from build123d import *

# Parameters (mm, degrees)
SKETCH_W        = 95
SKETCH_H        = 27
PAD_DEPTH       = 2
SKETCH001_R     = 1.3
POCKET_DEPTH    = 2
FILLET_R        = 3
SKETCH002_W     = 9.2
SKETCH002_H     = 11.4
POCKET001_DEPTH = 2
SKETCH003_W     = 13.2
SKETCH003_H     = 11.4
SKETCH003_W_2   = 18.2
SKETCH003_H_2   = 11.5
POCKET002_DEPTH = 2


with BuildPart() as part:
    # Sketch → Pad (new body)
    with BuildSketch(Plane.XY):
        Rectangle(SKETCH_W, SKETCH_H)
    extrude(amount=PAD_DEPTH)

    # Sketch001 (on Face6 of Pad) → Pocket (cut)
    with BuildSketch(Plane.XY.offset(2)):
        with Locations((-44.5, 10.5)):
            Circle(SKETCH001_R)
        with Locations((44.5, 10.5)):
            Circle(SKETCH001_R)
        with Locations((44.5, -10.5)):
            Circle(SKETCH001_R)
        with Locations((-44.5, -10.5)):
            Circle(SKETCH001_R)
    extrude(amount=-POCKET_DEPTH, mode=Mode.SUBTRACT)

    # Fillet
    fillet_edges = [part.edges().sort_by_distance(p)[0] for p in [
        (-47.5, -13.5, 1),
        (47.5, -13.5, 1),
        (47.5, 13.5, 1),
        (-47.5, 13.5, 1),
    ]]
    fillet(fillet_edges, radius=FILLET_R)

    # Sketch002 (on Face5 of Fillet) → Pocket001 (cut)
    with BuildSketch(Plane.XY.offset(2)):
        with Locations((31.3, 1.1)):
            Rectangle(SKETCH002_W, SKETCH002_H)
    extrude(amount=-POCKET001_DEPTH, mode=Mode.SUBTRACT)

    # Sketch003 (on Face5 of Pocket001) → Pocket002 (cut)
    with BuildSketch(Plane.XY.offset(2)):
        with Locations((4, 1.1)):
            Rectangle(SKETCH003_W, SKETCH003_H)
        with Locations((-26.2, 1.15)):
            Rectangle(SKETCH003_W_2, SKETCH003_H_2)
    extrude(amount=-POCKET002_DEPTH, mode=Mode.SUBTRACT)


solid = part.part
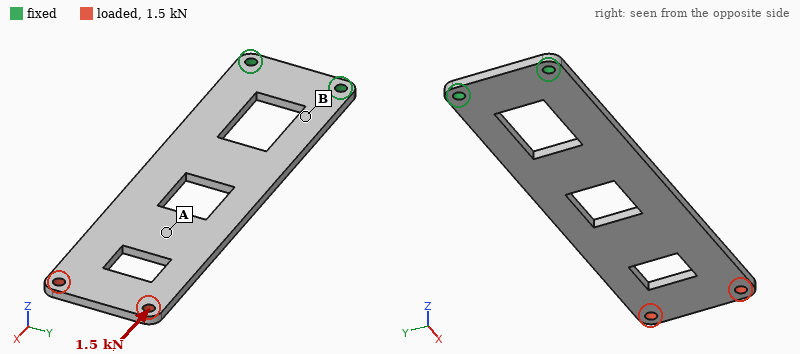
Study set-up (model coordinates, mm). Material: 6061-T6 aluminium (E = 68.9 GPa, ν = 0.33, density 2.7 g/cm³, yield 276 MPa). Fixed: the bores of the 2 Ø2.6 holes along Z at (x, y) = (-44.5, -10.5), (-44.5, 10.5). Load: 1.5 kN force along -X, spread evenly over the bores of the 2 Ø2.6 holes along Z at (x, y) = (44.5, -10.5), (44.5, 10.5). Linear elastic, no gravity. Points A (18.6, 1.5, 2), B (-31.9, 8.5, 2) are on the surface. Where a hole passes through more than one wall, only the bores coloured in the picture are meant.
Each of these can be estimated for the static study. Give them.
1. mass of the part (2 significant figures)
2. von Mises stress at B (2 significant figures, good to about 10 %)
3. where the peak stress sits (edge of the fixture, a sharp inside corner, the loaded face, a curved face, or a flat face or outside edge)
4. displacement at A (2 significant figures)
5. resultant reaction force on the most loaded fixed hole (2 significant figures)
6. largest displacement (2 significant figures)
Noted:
11 g
54 MPa
the loaded face
45 µm
760 N
72 µm
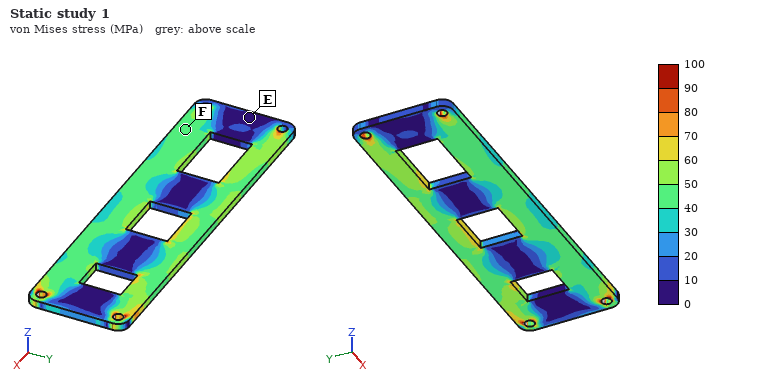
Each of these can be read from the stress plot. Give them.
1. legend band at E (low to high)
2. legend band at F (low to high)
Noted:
0 to 10 MPa
40 to 50 MPa
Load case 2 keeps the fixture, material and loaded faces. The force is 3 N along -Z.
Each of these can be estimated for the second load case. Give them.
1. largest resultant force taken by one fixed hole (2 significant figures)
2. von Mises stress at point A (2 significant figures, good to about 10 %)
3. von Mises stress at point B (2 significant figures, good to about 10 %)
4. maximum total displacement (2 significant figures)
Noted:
1.6 N
3.5 MPa
23 MPa
0.90 mm
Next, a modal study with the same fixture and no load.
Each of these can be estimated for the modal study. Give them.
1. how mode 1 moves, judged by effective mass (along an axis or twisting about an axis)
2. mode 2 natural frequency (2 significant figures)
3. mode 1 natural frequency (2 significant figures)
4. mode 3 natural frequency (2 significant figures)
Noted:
along Z
1100 Hz
170 Hz
1100 Hz
